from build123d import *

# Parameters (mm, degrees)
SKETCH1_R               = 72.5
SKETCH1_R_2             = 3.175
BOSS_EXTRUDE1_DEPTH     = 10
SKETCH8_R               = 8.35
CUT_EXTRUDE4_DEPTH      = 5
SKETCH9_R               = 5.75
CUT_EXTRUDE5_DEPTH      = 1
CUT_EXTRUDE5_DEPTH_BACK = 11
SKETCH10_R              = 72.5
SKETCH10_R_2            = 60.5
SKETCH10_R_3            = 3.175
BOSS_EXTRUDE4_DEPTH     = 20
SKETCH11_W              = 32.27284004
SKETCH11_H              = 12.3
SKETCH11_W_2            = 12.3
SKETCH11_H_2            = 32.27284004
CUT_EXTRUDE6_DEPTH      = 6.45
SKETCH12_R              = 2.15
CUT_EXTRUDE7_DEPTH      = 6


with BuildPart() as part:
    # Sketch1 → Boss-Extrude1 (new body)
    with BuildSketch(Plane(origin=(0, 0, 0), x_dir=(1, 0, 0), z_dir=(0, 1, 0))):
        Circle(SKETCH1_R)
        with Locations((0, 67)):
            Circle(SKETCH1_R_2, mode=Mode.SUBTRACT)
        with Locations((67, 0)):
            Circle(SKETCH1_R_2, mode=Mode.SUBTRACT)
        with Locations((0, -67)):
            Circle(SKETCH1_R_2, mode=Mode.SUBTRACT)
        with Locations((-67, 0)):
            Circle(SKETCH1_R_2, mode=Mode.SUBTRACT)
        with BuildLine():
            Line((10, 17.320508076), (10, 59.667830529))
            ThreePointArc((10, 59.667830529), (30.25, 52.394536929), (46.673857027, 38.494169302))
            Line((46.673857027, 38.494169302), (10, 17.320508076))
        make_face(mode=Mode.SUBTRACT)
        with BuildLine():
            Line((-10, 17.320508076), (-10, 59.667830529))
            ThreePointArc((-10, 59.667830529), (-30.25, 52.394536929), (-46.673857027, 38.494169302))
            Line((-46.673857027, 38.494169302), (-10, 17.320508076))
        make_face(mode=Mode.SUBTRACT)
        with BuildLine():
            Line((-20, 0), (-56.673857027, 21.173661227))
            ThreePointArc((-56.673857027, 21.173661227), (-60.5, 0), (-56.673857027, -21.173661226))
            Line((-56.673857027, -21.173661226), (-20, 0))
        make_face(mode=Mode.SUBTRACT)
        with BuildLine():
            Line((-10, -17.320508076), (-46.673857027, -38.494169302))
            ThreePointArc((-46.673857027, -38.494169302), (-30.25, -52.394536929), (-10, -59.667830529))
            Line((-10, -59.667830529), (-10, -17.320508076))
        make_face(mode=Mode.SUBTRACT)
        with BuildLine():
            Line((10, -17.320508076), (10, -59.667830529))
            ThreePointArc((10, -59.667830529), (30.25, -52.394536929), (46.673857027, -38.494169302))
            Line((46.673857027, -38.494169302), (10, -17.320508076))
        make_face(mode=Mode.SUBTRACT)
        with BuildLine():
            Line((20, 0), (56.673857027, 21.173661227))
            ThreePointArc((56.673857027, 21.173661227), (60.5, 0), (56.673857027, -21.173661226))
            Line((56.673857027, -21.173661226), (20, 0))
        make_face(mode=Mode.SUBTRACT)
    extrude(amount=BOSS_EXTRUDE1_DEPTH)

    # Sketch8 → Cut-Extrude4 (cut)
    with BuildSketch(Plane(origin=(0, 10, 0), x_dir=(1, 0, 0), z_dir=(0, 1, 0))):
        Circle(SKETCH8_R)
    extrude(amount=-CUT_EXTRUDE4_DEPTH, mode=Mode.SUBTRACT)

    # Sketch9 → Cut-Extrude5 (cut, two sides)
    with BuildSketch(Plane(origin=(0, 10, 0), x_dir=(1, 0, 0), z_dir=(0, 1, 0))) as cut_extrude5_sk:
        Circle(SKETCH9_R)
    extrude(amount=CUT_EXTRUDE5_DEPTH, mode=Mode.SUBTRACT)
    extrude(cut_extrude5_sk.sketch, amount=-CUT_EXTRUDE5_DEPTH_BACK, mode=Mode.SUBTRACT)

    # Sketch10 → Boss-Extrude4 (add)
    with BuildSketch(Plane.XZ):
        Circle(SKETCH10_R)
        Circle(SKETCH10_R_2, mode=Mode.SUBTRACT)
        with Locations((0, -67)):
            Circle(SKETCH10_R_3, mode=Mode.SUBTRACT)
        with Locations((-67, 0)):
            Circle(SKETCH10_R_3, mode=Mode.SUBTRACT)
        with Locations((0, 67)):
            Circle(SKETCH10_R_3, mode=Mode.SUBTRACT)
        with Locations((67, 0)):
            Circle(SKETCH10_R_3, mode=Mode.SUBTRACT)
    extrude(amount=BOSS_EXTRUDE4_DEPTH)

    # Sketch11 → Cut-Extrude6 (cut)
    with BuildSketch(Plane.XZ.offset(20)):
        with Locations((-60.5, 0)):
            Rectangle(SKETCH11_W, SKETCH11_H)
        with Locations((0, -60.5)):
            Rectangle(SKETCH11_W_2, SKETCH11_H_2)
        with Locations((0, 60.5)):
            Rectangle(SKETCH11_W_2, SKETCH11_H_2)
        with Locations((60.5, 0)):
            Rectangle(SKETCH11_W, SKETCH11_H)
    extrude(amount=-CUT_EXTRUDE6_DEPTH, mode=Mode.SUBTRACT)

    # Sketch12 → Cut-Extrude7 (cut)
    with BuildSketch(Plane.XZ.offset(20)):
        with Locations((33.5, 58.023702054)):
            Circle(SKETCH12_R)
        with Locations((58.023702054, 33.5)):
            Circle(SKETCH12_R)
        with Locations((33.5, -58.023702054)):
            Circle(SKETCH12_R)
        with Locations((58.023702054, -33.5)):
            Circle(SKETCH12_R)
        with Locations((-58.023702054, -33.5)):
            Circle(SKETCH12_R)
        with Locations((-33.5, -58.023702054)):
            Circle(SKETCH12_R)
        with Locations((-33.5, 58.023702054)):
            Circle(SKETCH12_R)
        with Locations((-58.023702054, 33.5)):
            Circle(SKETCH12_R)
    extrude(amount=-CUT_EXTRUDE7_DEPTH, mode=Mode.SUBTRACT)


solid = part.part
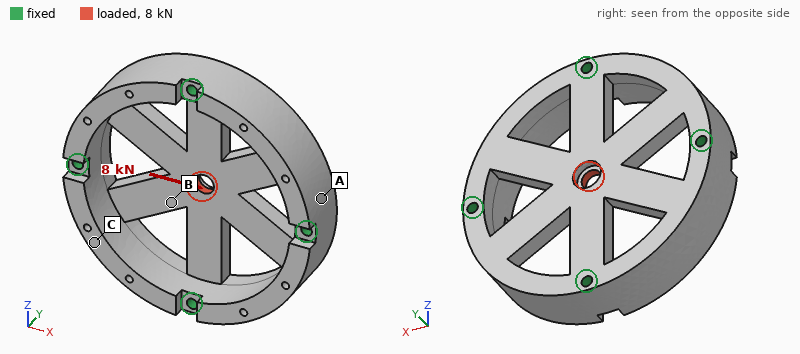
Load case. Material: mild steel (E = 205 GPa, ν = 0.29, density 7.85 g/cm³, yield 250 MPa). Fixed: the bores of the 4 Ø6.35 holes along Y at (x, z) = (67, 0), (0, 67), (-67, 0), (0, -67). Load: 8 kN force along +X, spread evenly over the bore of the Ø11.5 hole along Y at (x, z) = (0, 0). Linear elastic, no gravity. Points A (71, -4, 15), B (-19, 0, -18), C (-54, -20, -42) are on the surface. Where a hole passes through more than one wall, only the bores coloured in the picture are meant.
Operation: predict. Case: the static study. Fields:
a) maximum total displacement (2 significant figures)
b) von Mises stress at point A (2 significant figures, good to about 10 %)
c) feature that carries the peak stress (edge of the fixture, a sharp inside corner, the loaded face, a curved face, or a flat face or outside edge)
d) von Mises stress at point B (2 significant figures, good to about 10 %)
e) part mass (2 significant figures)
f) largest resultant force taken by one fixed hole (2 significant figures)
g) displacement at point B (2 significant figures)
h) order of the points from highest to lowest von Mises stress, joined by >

11 µm
10 MPa
a sharp inside corner
22 MPa
1.6 kg
2.8 kN
7.7 µm
B > A > C
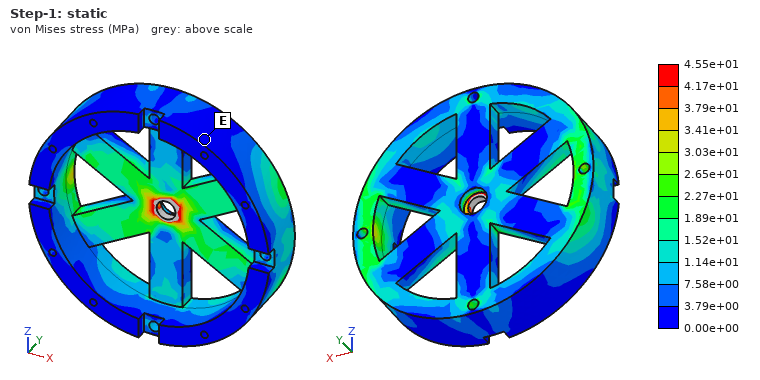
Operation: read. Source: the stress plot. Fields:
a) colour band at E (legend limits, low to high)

0.00e+00 to 3.79e+00 MPa
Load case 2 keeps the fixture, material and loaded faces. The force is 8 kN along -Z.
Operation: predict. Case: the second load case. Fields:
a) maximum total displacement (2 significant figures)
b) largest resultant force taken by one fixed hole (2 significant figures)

6.6 µm
2.8 kN
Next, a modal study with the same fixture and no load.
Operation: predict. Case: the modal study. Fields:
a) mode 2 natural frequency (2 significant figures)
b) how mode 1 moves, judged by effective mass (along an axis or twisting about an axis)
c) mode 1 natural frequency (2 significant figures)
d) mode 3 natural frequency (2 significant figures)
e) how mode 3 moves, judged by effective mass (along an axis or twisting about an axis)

7200 Hz
along Y
3700 Hz
7500 Hz
twisting about X
